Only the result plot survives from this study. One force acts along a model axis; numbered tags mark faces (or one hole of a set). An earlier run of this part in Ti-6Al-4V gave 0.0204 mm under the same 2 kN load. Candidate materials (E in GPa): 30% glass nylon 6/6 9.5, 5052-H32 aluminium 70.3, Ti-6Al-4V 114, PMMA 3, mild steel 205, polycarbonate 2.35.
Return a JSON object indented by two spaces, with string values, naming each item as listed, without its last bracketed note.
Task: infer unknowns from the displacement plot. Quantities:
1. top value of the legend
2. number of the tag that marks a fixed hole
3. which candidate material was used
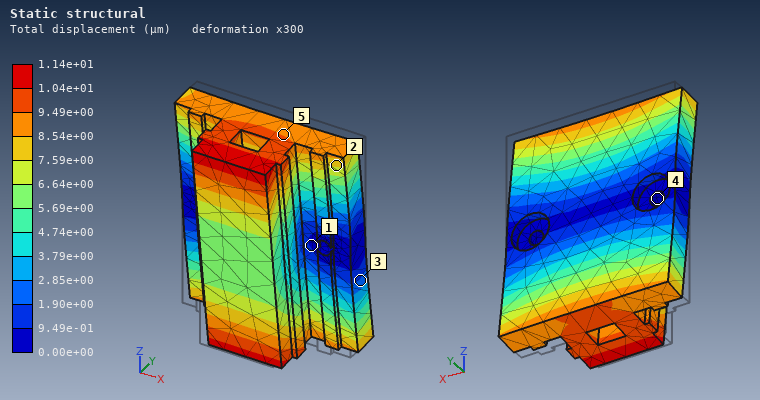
{
  "top value of the legend": "1.14e+01 µm",
  "number of the tag that marks a fixed hole": "4",
  "which candidate material was used": "mild steel"
}
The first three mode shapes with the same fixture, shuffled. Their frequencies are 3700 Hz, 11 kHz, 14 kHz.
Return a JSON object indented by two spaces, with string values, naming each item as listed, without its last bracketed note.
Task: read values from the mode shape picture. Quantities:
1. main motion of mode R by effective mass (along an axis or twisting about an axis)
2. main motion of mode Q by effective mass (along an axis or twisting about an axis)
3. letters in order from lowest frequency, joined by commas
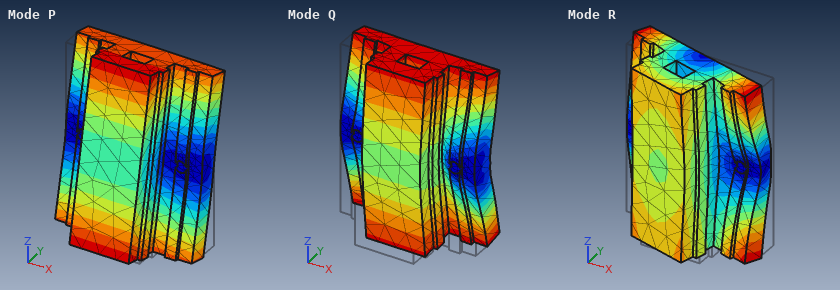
{
  "main motion of mode R by effective mass": "along X",
  "main motion of mode Q by effective mass": "along Y",
  "letters in order from lowest frequency, joined by commas": "P, Q, R"
}
